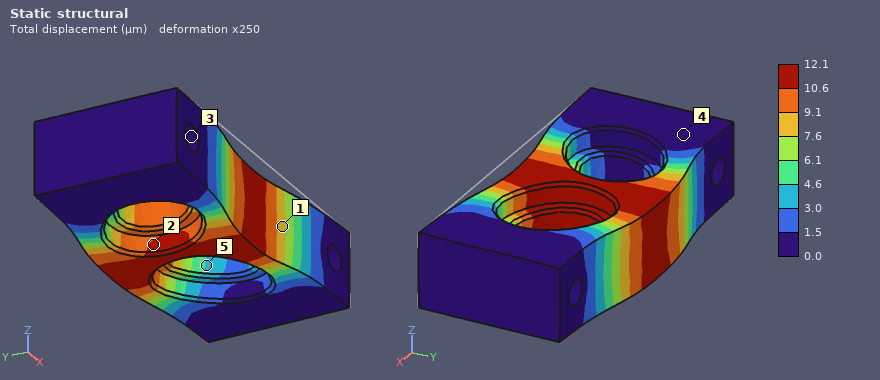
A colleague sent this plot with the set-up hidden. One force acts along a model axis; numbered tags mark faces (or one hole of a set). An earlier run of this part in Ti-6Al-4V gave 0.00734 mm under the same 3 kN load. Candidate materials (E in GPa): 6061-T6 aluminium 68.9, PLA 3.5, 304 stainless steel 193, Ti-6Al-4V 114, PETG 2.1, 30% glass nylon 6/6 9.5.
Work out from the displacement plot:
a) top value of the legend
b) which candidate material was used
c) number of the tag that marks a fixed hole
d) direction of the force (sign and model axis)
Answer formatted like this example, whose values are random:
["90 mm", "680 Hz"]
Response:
["12.1 µm", "6061-T6 aluminium", "3", "+Y"]
